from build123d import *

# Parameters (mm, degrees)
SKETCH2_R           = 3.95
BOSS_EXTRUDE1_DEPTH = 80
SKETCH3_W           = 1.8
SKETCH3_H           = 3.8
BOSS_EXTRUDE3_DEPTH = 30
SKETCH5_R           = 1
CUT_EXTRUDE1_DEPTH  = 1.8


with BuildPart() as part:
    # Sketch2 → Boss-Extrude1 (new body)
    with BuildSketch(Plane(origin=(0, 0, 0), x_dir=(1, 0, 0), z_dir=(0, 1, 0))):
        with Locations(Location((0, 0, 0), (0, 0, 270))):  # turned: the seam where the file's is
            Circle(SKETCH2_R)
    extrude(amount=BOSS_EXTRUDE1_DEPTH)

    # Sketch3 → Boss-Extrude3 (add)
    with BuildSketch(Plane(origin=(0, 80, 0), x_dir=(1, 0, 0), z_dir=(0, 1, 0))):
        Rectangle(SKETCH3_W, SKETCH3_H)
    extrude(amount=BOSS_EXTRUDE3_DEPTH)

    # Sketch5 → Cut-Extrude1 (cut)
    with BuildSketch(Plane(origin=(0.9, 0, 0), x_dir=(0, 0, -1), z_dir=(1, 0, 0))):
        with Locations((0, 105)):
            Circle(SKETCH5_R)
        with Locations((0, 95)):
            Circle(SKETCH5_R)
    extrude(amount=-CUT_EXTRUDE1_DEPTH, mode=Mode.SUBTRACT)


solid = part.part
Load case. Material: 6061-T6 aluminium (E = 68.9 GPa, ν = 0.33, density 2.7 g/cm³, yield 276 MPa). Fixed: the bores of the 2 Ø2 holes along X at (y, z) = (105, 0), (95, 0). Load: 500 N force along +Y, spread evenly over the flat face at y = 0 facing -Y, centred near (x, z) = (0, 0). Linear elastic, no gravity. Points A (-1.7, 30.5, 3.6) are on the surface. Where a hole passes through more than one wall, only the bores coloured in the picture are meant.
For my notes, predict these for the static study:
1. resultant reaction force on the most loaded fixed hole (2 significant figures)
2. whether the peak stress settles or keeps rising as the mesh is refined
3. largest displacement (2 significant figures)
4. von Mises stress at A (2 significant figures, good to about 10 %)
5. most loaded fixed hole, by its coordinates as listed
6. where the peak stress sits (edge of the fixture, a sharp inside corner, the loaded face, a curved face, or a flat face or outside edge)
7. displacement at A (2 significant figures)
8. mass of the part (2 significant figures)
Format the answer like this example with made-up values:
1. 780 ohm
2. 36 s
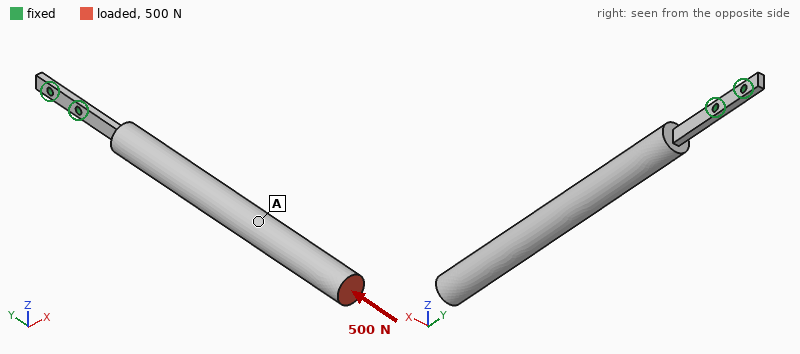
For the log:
1. 490 N
2. keeps rising
3. 28 µm
4. 10 MPa
5. (95, 0)
6. edge of the fixture
7. 24 µm
8. 11 g
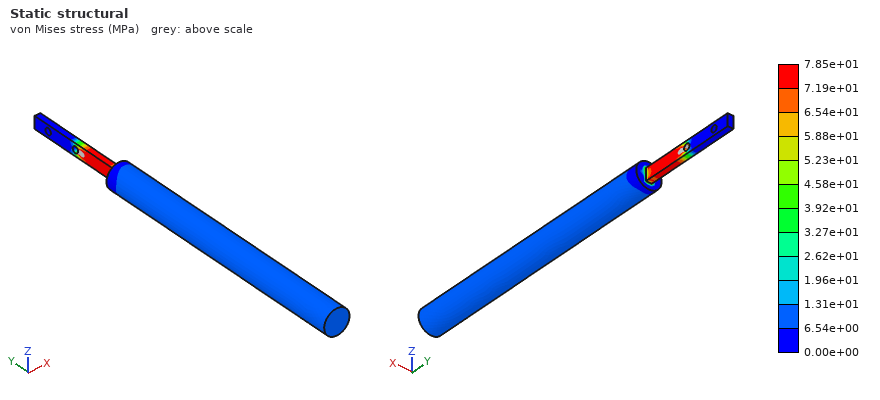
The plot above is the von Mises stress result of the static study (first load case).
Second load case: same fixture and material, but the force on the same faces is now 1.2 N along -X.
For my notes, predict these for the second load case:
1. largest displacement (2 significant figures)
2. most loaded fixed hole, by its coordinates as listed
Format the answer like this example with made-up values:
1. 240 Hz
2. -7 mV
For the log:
1. 1.1 mm
2. (95, 0)
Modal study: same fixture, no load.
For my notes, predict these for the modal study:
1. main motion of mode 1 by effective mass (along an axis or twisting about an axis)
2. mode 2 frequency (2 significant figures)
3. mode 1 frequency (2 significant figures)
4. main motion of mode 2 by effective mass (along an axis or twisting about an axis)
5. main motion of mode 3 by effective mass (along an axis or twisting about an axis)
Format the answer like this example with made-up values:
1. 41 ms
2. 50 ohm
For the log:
1. along X
2. 170 Hz
3. 86 Hz
4. along Z
5. twisting about Y
